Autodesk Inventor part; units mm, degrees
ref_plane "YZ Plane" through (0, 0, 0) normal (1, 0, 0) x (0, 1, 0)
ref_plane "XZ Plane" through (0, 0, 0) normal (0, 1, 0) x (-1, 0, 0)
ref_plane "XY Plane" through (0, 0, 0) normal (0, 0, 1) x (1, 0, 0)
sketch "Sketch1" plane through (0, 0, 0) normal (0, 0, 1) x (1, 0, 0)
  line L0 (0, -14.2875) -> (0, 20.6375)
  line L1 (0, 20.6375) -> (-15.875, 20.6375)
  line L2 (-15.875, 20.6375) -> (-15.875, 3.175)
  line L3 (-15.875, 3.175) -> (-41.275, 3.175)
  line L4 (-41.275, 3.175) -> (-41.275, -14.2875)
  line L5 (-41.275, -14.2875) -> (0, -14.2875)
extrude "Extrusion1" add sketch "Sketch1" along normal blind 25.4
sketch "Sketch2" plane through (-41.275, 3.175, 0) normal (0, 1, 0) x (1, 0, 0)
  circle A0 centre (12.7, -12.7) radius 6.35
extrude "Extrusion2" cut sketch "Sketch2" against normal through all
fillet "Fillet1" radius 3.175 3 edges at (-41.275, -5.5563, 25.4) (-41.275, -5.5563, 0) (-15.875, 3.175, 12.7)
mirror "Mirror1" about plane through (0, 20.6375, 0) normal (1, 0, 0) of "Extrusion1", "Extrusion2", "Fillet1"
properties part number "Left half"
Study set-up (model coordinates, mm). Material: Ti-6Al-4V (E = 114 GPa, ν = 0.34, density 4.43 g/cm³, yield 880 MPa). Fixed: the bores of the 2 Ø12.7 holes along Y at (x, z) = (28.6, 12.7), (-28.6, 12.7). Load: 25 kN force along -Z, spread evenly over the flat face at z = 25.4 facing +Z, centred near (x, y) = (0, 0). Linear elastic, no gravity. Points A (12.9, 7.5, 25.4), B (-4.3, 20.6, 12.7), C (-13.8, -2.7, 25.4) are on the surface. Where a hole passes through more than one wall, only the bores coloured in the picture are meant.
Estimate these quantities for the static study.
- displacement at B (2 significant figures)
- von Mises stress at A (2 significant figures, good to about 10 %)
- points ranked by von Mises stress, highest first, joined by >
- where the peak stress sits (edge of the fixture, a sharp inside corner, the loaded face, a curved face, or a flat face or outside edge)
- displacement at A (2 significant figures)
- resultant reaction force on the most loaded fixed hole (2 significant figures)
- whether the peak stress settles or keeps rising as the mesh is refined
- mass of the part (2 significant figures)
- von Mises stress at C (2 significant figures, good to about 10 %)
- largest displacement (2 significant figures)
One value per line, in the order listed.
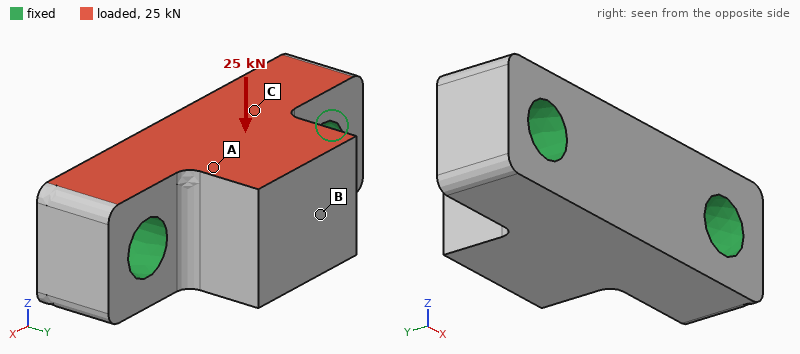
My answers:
31 µm
24 MPa
C > A > B
edge of the fixture
22 µm
13 kN
keeps rising
200 g
51 MPa
35 µm
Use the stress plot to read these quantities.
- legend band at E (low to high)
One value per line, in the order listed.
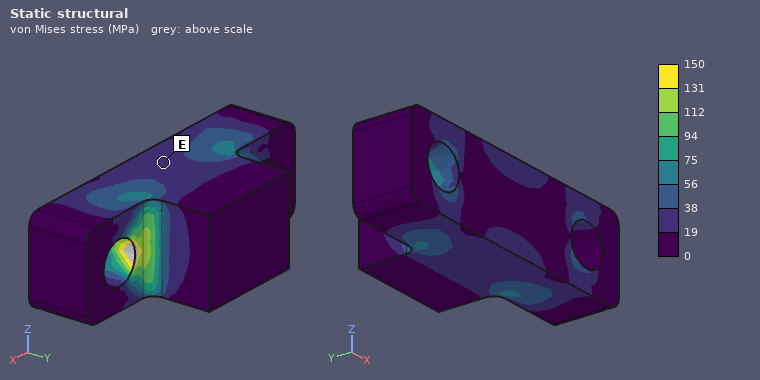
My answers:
19 to 38 MPa
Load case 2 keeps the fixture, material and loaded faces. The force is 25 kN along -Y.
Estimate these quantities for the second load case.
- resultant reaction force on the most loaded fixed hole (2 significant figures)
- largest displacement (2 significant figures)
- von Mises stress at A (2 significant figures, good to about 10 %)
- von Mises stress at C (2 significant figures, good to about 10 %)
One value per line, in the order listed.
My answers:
13 kN
45 µm
53 MPa
77 MPa
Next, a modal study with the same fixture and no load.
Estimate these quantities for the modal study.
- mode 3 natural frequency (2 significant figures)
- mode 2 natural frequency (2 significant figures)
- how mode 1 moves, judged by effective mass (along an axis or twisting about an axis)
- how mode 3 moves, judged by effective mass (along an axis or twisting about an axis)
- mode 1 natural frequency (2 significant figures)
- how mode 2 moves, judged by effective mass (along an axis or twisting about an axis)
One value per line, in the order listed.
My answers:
23 kHz
20 kHz
along Z
along X
11 kHz
along Y
